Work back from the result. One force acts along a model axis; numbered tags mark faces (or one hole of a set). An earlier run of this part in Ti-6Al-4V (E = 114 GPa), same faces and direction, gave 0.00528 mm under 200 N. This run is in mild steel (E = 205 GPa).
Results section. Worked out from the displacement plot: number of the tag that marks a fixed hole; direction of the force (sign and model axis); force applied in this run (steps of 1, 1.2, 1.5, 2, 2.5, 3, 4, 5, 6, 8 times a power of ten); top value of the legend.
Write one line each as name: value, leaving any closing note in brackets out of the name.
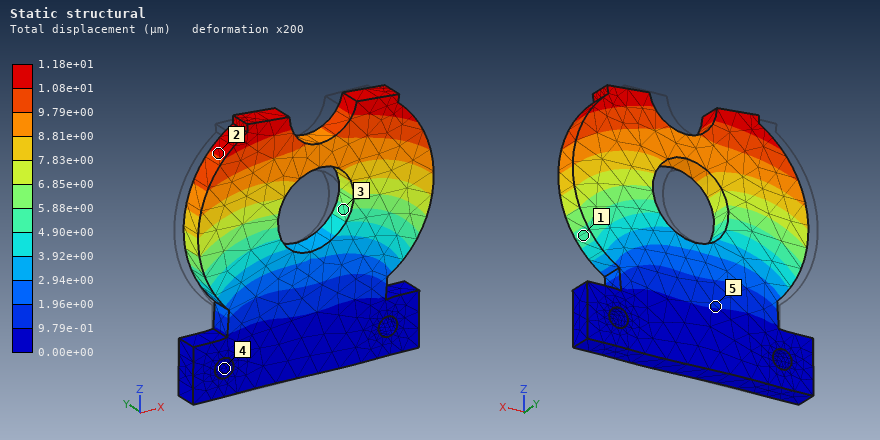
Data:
number of the tag that marks a fixed hole: 4
direction of the force: +X
force applied in this run: 800 N
top value of the legend: 1.18e+01 µm
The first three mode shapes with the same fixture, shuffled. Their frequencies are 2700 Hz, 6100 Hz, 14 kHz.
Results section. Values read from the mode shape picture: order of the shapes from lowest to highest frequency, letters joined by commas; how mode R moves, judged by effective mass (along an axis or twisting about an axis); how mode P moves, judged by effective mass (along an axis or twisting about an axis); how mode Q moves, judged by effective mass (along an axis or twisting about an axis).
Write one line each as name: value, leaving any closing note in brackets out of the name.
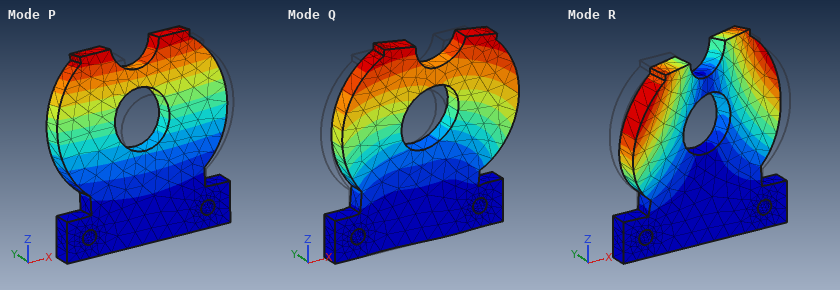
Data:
order of the shapes from lowest to highest frequency, letters joined by commas: P, R, Q
how mode R moves, judged by effective mass: twisting about Z
how mode P moves, judged by effective mass: along Y
how mode Q moves, judged by effective mass: along X
